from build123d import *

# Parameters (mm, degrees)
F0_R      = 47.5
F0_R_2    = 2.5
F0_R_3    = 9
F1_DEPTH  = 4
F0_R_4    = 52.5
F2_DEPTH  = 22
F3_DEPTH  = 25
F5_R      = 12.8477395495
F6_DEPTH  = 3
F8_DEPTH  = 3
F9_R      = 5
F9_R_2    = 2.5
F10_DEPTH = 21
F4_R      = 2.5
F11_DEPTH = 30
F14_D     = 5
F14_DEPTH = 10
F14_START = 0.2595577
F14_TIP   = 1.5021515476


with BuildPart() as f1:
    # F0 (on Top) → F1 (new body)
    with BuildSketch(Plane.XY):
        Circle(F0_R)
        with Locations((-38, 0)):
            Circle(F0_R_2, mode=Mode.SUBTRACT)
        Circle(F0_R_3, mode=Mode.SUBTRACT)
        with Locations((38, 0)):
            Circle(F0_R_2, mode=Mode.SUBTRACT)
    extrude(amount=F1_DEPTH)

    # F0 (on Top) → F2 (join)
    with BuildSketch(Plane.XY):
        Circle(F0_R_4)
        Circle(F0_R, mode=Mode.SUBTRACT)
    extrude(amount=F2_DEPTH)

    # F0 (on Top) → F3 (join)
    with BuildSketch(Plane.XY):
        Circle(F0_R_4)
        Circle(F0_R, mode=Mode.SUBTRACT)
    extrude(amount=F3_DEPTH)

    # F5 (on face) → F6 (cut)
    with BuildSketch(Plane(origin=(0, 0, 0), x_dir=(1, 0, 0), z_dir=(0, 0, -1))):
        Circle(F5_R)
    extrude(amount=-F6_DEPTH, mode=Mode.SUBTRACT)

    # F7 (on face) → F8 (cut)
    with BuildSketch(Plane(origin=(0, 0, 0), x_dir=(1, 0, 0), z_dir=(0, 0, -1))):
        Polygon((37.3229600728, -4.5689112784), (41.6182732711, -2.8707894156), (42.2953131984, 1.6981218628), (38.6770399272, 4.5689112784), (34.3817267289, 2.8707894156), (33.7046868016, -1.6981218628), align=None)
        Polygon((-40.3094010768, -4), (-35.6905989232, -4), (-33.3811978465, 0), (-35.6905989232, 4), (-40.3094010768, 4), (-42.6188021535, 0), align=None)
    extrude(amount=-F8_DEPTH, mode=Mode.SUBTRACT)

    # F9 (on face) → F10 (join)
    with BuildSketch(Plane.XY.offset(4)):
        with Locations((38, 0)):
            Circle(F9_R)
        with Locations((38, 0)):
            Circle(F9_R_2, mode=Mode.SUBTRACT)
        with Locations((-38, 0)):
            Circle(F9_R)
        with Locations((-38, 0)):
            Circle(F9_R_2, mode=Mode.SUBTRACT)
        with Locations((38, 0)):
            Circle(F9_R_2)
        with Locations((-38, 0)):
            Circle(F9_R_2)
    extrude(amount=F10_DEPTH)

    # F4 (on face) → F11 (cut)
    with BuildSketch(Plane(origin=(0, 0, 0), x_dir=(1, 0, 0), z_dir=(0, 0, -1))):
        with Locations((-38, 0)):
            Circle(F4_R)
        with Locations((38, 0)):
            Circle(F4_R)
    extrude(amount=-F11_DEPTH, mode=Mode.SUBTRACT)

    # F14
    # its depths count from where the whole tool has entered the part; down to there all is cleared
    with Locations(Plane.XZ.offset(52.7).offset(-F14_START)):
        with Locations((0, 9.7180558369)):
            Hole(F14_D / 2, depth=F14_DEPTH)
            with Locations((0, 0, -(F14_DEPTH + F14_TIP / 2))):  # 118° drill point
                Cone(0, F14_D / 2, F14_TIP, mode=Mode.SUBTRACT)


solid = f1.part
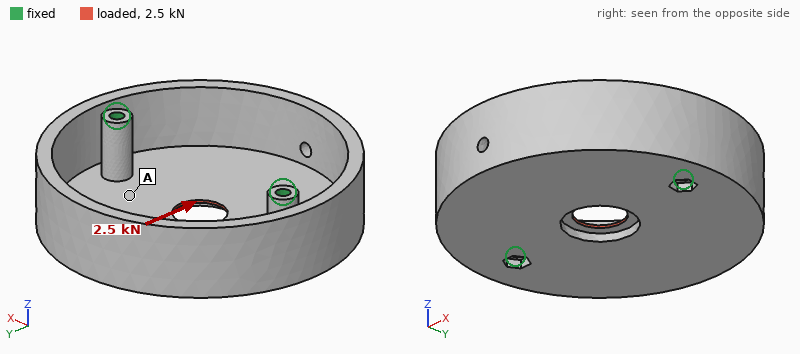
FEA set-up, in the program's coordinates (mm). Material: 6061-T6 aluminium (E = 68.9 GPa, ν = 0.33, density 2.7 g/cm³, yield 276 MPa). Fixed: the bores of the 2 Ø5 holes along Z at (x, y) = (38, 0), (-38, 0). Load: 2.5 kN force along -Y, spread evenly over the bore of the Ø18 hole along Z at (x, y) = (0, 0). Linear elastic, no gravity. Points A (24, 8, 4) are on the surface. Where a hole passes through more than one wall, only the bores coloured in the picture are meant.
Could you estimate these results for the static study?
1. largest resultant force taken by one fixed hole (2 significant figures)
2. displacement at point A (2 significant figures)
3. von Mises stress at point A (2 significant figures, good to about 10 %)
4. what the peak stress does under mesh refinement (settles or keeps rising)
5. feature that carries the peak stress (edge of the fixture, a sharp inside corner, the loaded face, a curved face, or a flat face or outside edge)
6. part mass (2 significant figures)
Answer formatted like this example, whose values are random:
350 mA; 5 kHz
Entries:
1.3 kN; 5.8 µm; 9.2 MPa; keeps rising; a sharp inside corner; 180 g
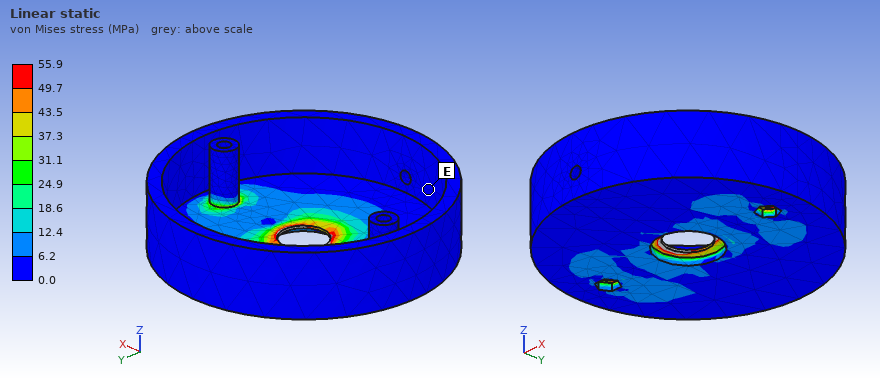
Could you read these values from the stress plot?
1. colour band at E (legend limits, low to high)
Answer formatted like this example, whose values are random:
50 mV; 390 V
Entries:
0.0 to 6.2 MPa
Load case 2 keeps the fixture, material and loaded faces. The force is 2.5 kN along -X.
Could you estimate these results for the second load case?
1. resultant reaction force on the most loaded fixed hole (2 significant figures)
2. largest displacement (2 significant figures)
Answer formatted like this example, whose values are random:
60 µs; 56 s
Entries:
1.3 kN; 13 µm
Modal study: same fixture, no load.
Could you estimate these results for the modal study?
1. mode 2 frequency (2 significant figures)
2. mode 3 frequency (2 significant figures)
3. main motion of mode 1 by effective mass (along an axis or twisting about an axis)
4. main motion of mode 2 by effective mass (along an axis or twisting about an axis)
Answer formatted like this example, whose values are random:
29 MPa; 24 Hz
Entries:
2200 Hz; 2700 Hz; twisting about X; along Z
